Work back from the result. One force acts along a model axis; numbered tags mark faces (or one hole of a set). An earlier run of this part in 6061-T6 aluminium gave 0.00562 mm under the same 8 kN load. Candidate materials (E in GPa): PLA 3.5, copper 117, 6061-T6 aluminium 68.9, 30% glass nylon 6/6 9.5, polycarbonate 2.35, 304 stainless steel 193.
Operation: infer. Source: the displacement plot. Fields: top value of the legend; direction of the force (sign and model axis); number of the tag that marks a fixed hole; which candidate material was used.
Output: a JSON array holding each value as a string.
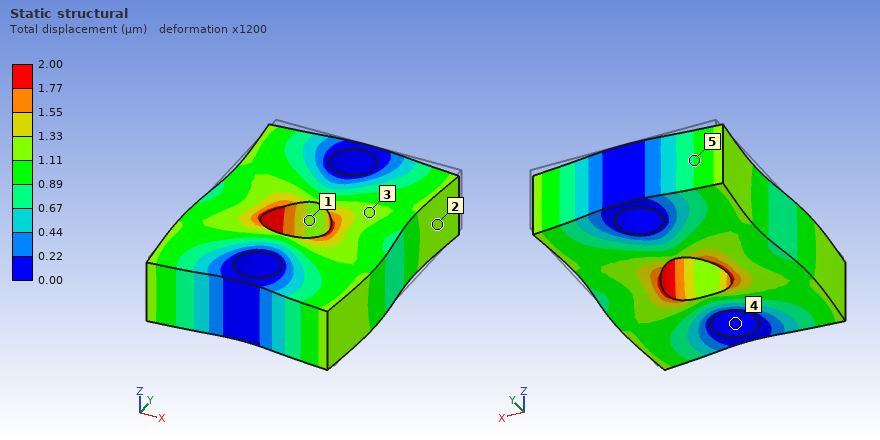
["2.00 µm", "-Y", "4", "304 stainless steel"]
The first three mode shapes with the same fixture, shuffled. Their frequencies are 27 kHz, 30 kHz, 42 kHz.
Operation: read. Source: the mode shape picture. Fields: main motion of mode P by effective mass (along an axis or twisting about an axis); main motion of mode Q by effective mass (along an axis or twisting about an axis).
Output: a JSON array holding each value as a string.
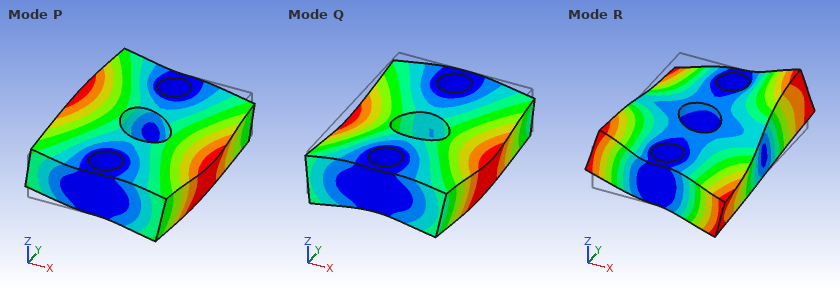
["twisting about Y", "along Z"]
